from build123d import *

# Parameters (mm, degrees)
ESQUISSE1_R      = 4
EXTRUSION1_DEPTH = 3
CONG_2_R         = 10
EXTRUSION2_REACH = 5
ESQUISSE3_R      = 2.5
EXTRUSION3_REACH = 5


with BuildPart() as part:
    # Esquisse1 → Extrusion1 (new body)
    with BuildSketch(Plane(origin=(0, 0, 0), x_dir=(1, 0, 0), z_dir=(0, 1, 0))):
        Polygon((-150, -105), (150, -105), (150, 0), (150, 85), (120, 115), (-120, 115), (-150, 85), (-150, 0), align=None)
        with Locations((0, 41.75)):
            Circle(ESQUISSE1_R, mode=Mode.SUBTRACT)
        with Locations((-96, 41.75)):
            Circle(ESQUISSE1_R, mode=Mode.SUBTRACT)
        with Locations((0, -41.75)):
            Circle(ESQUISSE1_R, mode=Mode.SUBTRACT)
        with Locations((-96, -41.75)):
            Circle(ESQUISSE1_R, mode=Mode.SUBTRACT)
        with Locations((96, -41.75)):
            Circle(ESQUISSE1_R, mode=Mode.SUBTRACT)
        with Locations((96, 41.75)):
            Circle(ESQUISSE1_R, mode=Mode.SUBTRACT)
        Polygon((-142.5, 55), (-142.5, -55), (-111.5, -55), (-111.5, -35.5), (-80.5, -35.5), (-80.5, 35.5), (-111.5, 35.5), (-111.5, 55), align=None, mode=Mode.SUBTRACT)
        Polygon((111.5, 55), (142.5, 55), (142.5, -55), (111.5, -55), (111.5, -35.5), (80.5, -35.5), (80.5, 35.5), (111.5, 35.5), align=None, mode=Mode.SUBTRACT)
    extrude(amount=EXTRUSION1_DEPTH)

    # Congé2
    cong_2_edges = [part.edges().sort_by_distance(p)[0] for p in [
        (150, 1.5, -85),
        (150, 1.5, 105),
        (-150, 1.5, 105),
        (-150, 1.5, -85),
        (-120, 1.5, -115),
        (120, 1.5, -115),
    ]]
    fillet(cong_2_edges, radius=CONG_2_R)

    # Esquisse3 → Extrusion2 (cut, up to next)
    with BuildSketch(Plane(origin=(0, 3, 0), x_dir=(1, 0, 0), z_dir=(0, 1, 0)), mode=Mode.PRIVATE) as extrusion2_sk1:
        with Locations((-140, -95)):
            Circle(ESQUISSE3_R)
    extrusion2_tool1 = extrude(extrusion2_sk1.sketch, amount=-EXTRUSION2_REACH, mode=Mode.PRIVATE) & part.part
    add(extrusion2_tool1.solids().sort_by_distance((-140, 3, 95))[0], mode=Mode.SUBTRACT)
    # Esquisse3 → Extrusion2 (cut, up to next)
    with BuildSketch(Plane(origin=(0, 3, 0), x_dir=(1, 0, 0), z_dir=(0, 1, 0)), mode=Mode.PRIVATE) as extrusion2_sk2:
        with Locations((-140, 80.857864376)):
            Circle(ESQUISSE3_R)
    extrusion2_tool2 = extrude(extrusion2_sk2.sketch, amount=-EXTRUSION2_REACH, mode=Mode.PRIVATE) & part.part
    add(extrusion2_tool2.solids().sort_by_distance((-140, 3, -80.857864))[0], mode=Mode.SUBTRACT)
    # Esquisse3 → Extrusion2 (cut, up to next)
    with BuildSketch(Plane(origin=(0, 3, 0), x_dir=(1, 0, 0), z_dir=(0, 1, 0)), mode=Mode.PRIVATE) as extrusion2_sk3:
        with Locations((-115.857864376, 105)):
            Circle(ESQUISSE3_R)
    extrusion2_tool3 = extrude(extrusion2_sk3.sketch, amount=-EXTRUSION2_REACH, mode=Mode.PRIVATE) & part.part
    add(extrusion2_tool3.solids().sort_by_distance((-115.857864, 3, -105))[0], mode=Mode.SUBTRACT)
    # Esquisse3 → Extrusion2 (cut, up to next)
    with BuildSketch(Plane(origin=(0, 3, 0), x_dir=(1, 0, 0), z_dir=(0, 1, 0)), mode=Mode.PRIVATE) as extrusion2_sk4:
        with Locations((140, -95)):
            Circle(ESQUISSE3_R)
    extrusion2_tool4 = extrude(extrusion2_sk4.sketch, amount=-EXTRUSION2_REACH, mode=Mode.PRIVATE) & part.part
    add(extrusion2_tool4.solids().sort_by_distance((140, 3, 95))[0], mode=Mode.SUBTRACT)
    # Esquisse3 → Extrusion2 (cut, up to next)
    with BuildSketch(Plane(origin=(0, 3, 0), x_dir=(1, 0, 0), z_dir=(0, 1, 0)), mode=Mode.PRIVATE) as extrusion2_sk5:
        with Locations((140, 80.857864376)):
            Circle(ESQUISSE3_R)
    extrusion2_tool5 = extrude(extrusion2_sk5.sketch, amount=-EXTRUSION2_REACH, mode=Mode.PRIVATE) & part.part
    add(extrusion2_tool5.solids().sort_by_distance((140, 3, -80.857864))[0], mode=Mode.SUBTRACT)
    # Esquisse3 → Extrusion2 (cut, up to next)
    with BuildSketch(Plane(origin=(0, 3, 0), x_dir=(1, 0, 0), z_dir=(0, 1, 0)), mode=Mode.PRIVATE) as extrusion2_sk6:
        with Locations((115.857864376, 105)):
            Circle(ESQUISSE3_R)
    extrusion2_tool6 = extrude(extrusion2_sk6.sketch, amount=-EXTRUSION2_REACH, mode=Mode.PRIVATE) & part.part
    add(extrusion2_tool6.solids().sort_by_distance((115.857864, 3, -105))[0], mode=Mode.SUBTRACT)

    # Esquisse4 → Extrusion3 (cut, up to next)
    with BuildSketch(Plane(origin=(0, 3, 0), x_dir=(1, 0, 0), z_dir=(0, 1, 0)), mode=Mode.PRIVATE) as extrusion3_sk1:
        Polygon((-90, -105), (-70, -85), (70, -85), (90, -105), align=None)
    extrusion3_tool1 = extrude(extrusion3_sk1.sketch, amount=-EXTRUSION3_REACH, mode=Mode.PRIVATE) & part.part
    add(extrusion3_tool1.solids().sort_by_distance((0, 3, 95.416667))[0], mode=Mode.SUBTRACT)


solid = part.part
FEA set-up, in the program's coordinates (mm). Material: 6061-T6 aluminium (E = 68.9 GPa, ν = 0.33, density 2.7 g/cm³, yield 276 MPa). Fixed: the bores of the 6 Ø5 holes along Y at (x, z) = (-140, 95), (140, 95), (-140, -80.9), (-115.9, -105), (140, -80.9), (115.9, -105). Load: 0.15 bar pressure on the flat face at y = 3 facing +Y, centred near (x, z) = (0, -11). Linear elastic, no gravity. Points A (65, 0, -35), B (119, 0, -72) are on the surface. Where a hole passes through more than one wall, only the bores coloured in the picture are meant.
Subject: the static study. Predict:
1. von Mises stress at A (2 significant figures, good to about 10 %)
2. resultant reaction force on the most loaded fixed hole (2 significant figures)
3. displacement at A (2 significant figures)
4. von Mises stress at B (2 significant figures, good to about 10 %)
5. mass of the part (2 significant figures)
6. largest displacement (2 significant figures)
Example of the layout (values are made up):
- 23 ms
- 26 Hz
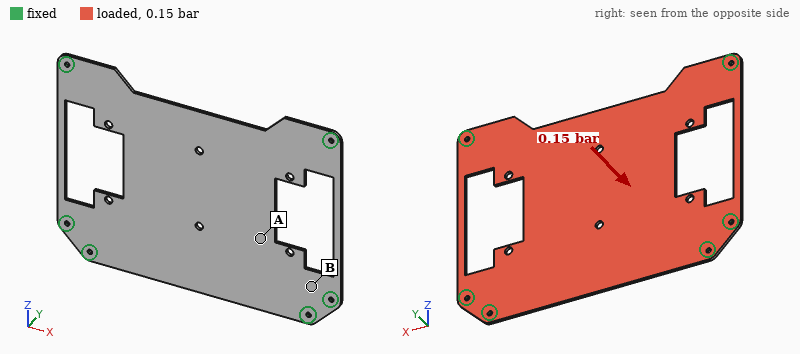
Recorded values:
- 18 MPa
- 180 N
- 1.4 mm
- 43 MPa
- 410 g
- 2.3 mm
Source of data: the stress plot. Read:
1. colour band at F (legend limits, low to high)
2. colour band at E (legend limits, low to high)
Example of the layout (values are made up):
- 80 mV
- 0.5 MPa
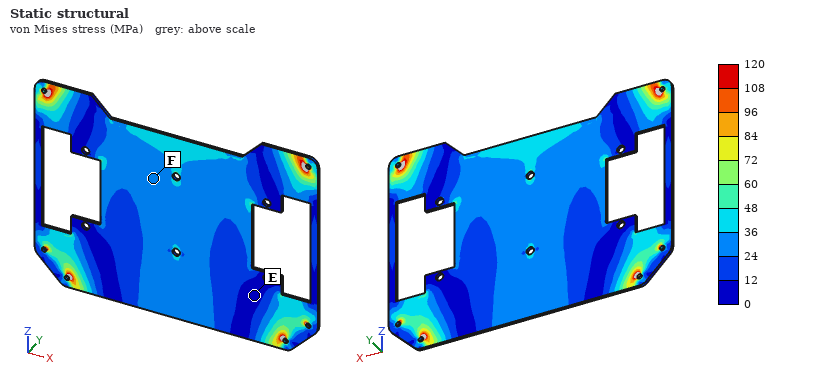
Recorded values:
- 24 to 36 MPa
- 0 to 12 MPa
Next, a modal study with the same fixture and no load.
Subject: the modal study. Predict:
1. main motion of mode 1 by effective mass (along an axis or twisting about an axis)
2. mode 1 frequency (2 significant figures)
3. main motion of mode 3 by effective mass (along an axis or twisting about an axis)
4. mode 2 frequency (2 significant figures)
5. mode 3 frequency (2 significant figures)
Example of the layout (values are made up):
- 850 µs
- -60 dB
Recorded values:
- along Y
- 170 Hz
- twisting about Z
- 310 Hz
- 420 Hz
